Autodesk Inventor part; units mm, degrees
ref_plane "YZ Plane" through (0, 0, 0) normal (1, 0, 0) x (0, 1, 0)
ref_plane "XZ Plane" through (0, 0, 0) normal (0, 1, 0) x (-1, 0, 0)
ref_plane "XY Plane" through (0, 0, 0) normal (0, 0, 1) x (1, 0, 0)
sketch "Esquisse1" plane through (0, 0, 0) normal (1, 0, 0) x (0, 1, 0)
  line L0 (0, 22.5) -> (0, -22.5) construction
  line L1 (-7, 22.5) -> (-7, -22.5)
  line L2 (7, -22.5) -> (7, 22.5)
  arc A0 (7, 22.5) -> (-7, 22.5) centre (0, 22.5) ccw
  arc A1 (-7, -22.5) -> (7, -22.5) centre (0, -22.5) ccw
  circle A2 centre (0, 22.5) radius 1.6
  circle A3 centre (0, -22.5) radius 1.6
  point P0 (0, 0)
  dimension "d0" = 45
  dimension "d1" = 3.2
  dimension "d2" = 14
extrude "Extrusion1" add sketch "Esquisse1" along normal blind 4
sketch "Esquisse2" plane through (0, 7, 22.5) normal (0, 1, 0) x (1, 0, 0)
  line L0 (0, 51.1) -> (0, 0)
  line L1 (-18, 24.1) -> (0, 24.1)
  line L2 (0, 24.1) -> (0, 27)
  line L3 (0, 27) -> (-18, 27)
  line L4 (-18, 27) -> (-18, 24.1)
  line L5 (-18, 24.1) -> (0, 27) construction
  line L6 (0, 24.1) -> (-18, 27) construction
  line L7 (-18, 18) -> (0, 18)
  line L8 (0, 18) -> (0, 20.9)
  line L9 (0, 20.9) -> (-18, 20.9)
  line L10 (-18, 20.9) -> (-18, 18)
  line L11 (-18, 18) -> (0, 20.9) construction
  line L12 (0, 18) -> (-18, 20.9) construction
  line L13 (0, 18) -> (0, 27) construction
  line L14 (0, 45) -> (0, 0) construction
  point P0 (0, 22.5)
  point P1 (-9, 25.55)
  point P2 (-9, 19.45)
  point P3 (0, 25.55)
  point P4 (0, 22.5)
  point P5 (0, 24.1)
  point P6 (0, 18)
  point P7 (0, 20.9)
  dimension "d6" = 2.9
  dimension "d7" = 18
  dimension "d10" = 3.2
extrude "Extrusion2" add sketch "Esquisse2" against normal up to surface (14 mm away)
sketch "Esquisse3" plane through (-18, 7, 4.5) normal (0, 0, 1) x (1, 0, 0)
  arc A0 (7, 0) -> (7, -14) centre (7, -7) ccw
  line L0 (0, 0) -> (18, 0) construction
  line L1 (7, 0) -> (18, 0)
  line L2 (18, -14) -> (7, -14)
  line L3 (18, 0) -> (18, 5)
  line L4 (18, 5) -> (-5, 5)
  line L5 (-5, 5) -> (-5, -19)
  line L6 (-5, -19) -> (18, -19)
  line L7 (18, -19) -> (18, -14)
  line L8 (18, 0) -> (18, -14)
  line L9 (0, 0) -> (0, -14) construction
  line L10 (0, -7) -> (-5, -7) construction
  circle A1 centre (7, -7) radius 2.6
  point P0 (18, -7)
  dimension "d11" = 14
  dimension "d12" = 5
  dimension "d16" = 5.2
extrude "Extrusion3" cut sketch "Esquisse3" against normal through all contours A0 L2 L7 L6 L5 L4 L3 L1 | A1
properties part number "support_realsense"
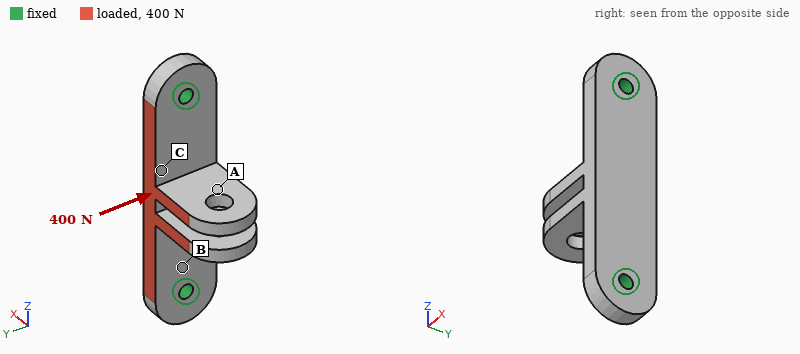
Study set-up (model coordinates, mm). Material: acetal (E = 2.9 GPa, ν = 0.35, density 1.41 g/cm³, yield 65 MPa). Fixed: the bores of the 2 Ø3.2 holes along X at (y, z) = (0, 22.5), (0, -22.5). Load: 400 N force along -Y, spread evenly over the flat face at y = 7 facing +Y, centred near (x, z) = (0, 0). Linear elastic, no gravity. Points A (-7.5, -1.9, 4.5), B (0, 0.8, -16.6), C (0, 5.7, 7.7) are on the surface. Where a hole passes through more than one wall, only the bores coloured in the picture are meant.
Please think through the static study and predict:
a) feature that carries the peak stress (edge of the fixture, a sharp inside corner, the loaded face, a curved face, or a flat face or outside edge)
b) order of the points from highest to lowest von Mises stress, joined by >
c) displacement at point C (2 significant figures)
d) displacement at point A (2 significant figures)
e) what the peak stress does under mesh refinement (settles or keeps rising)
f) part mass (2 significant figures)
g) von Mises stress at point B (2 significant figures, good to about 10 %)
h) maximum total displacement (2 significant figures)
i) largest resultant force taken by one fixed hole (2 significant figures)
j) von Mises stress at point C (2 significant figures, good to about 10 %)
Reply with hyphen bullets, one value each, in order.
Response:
- edge of the fixture
- B > C > A
- 0.21 mm
- 0.40 mm
- keeps rising
- 6.0 g
- 17 MPa
- 0.68 mm
- 200 N
- 10.0 MPa
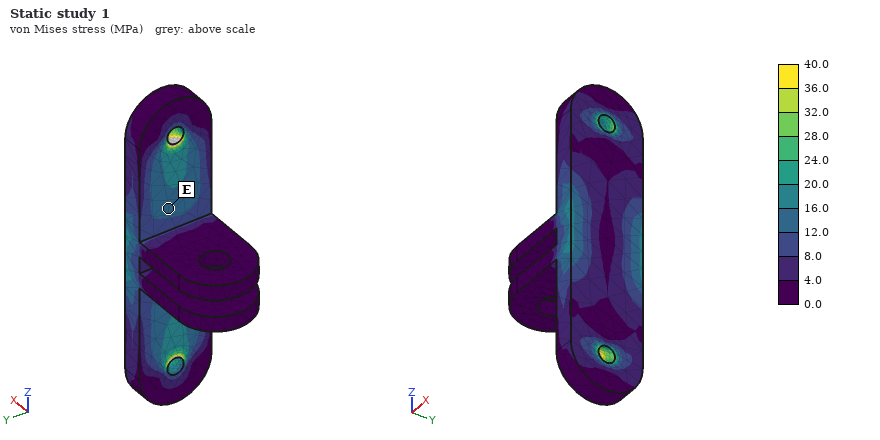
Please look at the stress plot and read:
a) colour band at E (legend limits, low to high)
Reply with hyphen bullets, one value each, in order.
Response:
- 12.0 to 16.0 MPa
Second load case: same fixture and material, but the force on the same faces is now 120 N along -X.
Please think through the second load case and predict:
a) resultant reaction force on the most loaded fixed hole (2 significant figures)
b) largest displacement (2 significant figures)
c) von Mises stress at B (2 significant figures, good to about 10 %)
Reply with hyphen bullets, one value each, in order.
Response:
- 60 N
- 0.44 mm
- 9.5 MPa
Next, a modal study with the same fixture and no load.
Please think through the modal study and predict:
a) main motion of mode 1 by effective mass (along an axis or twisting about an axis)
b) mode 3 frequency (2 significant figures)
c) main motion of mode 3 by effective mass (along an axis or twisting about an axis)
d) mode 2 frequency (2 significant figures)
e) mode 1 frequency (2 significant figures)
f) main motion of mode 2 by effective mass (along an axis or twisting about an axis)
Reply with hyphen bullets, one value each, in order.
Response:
- along Y
- 2000 Hz
- along Z
- 1800 Hz
- 1600 Hz
- along X
